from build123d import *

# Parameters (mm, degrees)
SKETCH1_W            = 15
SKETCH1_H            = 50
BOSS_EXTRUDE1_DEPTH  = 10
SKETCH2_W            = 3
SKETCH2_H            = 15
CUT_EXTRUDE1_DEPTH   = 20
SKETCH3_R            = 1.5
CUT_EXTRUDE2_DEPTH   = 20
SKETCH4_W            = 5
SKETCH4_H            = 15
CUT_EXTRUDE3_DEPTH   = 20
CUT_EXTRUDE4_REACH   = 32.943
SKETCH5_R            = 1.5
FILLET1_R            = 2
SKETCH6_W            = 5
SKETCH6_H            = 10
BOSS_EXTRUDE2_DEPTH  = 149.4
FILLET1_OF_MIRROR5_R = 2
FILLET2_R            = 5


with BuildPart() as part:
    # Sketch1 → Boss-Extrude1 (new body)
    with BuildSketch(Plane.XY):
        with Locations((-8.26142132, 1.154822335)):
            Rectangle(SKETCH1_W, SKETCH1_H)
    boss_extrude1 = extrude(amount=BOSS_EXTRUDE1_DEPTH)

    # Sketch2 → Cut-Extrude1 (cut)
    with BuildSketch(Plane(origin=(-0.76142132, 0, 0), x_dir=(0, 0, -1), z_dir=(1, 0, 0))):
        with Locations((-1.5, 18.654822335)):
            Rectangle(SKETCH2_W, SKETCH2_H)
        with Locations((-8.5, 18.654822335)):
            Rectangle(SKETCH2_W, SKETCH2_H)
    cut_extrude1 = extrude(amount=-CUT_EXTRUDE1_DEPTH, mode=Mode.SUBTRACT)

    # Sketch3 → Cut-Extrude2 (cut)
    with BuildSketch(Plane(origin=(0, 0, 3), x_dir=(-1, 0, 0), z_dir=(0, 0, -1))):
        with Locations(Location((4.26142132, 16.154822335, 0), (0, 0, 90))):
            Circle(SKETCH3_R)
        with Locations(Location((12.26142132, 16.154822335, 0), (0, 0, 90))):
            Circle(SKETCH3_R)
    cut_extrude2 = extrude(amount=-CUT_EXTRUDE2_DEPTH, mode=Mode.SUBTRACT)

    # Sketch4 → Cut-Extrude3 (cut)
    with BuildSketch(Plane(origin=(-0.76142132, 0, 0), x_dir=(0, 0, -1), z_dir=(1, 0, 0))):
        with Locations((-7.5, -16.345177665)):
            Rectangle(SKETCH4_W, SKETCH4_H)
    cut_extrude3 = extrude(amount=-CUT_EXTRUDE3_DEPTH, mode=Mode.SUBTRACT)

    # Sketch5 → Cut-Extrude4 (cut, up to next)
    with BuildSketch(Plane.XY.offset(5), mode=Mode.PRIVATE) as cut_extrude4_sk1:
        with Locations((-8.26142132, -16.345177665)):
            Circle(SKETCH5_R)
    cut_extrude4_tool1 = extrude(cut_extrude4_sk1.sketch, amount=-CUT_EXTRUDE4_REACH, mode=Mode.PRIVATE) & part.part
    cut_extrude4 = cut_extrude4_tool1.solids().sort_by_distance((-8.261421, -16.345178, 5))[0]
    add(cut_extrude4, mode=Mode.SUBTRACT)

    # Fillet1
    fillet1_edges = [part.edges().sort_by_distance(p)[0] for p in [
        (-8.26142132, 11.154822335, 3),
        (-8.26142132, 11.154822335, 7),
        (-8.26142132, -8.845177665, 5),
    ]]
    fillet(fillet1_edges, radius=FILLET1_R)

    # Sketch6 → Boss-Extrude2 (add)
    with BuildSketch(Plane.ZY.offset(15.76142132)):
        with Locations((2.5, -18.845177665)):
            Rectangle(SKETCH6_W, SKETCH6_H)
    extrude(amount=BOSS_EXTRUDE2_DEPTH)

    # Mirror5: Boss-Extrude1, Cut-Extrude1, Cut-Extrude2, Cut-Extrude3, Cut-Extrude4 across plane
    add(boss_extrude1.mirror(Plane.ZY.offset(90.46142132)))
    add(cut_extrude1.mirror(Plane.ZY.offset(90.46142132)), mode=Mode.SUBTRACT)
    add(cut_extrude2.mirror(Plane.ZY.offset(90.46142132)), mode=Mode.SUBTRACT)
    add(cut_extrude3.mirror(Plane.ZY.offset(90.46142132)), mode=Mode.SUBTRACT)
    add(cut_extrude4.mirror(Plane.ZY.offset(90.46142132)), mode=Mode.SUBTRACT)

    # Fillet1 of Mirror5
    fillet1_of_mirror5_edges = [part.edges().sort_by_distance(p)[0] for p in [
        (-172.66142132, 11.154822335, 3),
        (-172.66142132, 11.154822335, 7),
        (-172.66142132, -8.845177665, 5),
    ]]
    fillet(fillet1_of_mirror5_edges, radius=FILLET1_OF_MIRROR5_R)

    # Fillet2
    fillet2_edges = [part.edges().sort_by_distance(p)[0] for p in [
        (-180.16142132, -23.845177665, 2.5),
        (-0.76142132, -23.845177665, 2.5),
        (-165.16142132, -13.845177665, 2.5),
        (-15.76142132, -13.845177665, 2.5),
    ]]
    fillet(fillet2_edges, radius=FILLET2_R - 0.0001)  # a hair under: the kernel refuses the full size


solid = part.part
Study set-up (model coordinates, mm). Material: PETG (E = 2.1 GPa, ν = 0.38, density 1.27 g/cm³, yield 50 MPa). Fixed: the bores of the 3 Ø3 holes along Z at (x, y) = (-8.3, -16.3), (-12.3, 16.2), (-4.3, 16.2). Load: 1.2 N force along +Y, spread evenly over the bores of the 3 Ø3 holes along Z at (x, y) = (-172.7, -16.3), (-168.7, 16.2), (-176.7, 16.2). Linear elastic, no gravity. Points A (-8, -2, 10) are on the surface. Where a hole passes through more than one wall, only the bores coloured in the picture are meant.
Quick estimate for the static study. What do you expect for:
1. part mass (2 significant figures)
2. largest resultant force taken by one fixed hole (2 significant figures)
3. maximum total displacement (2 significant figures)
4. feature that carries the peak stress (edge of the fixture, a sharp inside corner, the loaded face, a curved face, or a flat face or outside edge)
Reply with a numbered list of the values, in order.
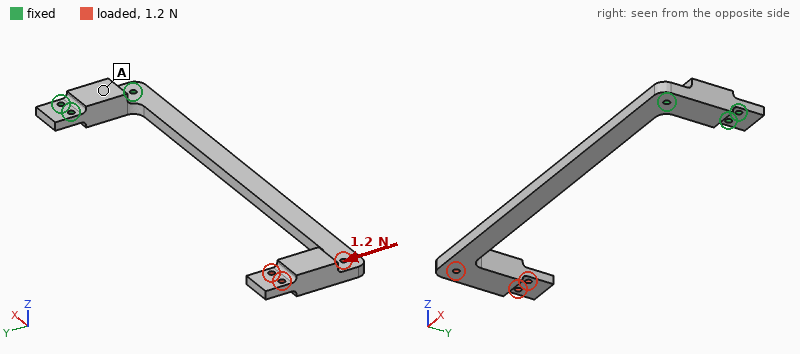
1. 22 g
2. 6.5 N
3. 2.2 mm
4. a curved face
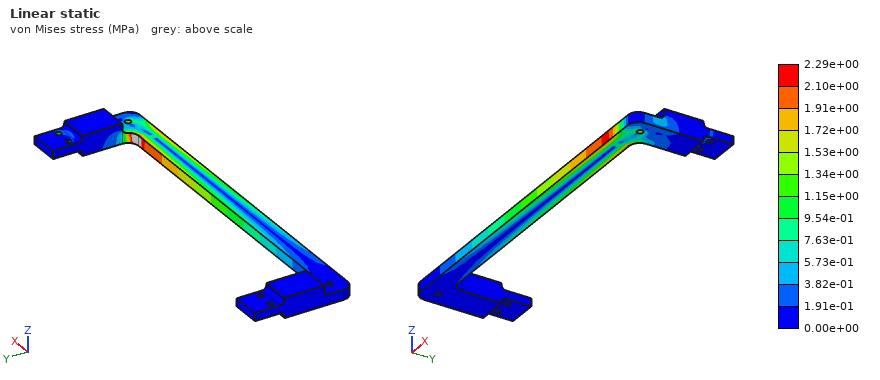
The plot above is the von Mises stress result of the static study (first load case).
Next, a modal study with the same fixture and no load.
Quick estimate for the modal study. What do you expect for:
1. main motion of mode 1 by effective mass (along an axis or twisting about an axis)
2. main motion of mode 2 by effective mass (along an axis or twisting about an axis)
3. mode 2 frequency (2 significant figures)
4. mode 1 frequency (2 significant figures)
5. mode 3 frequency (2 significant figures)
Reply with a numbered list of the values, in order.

1. along Z
2. along Y
3. 43 Hz
4. 21 Hz
5. 140 Hz
